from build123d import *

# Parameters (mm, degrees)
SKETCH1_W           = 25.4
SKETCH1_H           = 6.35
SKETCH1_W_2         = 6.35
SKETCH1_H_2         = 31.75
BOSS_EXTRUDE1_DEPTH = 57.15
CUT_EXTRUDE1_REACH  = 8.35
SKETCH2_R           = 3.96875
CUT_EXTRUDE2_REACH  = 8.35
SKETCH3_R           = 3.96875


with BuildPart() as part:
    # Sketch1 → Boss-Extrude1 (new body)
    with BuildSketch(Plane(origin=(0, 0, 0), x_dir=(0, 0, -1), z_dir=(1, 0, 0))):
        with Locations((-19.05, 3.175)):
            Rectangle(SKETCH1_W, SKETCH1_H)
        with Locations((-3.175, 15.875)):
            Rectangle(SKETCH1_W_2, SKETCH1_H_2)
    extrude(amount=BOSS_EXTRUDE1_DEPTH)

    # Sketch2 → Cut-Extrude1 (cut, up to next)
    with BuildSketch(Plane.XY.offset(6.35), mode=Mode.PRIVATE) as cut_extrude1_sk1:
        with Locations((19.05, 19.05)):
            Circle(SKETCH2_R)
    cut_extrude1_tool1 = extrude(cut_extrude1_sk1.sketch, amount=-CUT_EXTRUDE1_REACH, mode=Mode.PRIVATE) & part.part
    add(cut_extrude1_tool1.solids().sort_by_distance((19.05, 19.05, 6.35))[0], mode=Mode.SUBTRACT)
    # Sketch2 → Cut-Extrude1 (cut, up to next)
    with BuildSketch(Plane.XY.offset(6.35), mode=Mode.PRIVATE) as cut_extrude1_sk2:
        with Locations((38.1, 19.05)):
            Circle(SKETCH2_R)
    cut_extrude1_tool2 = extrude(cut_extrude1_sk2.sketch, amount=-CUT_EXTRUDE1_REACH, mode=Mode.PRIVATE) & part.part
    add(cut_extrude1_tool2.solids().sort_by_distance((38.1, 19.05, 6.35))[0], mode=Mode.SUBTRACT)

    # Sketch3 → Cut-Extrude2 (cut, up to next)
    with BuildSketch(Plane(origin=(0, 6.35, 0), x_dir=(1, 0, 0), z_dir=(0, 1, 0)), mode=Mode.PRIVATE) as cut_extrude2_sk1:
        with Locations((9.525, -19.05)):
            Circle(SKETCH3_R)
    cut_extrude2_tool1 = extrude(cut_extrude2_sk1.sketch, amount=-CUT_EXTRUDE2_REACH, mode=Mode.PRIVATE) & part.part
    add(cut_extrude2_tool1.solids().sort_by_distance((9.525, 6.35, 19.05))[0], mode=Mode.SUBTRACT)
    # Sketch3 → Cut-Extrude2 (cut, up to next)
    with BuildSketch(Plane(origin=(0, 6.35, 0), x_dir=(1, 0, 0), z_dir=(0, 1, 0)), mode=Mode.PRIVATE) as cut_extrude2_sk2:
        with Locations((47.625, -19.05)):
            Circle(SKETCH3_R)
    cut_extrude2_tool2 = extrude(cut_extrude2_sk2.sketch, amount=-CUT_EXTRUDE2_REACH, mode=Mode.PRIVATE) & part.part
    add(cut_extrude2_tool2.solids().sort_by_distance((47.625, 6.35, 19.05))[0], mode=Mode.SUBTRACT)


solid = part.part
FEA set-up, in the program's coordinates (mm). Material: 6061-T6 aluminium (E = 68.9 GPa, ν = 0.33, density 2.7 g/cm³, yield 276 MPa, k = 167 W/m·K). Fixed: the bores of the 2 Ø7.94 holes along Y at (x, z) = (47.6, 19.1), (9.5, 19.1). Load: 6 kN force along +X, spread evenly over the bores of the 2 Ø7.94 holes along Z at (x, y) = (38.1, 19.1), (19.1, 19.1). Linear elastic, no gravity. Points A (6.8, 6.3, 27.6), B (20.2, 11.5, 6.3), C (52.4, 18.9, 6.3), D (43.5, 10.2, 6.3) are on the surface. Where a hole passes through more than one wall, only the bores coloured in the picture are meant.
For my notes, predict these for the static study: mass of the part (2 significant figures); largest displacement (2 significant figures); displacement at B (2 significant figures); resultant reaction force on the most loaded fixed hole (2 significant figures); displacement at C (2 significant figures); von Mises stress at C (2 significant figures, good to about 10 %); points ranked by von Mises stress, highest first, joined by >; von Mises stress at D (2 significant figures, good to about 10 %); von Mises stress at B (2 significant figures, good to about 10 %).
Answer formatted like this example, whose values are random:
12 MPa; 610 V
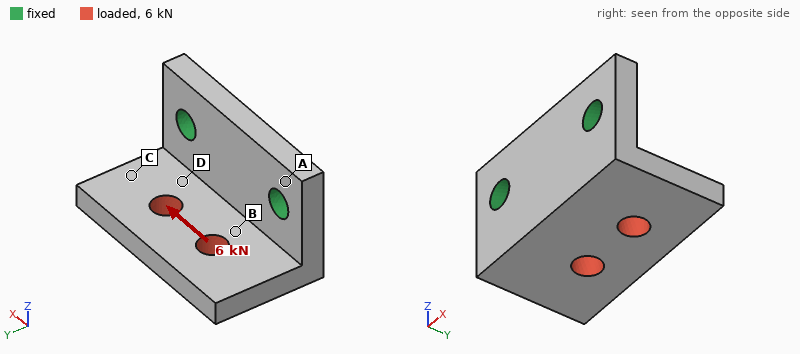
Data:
53 g; 0.13 mm; 0.039 mm; 4.3 kN; 0.082 mm; 32 MPa; B > D > C > A; 64 MPa; 85 MPa
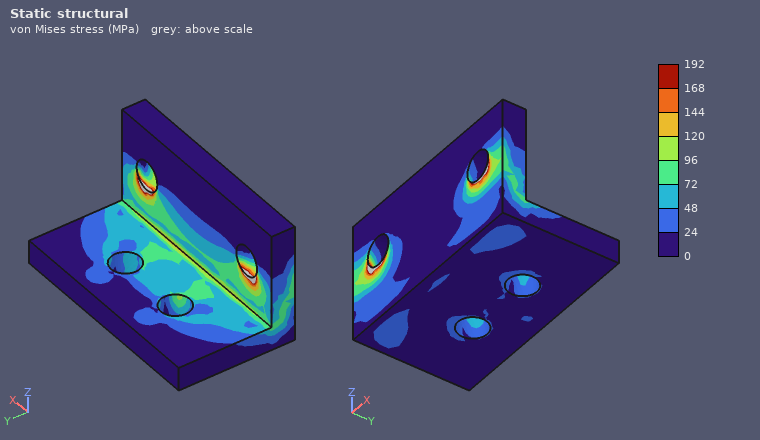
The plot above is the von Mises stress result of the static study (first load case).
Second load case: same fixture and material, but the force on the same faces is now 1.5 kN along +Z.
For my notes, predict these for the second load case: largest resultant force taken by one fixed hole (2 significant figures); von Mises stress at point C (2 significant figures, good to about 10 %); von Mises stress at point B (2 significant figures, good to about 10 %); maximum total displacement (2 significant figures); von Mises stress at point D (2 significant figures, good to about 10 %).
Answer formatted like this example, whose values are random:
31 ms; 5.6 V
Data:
780 N; 11 MPa; 26 MPa; 0.17 mm; 31 MPa
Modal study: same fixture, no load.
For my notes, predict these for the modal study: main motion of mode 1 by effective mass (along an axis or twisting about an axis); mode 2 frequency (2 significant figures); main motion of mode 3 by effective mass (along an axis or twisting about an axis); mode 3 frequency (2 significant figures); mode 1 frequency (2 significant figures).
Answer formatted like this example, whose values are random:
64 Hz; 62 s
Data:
along Z; 6300 Hz; along X; 9900 Hz; 3600 Hz
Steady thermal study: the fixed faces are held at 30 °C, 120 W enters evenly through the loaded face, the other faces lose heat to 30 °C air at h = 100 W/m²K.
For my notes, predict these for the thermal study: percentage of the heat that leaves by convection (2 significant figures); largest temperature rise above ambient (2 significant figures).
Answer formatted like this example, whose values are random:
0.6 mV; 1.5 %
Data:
17 %; 63 K
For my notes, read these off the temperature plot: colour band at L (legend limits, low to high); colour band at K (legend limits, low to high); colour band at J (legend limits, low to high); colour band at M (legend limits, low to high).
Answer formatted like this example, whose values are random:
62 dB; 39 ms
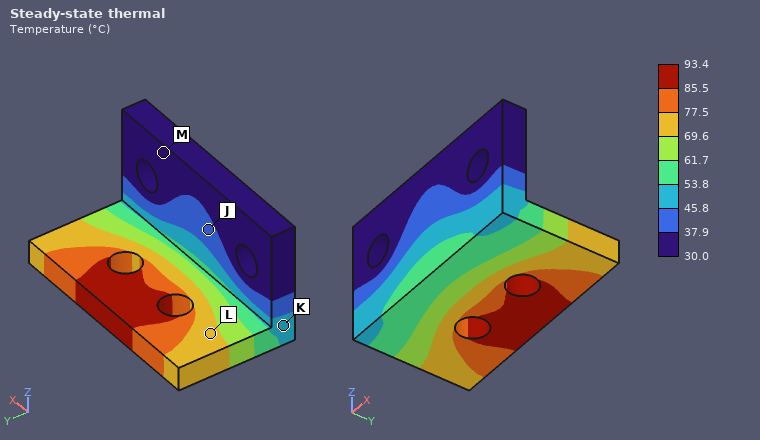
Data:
69.6 to 77.5 °C; 45.8 to 53.8 °C; 37.9 to 45.8 °C; 30.0 to 37.9 °C
